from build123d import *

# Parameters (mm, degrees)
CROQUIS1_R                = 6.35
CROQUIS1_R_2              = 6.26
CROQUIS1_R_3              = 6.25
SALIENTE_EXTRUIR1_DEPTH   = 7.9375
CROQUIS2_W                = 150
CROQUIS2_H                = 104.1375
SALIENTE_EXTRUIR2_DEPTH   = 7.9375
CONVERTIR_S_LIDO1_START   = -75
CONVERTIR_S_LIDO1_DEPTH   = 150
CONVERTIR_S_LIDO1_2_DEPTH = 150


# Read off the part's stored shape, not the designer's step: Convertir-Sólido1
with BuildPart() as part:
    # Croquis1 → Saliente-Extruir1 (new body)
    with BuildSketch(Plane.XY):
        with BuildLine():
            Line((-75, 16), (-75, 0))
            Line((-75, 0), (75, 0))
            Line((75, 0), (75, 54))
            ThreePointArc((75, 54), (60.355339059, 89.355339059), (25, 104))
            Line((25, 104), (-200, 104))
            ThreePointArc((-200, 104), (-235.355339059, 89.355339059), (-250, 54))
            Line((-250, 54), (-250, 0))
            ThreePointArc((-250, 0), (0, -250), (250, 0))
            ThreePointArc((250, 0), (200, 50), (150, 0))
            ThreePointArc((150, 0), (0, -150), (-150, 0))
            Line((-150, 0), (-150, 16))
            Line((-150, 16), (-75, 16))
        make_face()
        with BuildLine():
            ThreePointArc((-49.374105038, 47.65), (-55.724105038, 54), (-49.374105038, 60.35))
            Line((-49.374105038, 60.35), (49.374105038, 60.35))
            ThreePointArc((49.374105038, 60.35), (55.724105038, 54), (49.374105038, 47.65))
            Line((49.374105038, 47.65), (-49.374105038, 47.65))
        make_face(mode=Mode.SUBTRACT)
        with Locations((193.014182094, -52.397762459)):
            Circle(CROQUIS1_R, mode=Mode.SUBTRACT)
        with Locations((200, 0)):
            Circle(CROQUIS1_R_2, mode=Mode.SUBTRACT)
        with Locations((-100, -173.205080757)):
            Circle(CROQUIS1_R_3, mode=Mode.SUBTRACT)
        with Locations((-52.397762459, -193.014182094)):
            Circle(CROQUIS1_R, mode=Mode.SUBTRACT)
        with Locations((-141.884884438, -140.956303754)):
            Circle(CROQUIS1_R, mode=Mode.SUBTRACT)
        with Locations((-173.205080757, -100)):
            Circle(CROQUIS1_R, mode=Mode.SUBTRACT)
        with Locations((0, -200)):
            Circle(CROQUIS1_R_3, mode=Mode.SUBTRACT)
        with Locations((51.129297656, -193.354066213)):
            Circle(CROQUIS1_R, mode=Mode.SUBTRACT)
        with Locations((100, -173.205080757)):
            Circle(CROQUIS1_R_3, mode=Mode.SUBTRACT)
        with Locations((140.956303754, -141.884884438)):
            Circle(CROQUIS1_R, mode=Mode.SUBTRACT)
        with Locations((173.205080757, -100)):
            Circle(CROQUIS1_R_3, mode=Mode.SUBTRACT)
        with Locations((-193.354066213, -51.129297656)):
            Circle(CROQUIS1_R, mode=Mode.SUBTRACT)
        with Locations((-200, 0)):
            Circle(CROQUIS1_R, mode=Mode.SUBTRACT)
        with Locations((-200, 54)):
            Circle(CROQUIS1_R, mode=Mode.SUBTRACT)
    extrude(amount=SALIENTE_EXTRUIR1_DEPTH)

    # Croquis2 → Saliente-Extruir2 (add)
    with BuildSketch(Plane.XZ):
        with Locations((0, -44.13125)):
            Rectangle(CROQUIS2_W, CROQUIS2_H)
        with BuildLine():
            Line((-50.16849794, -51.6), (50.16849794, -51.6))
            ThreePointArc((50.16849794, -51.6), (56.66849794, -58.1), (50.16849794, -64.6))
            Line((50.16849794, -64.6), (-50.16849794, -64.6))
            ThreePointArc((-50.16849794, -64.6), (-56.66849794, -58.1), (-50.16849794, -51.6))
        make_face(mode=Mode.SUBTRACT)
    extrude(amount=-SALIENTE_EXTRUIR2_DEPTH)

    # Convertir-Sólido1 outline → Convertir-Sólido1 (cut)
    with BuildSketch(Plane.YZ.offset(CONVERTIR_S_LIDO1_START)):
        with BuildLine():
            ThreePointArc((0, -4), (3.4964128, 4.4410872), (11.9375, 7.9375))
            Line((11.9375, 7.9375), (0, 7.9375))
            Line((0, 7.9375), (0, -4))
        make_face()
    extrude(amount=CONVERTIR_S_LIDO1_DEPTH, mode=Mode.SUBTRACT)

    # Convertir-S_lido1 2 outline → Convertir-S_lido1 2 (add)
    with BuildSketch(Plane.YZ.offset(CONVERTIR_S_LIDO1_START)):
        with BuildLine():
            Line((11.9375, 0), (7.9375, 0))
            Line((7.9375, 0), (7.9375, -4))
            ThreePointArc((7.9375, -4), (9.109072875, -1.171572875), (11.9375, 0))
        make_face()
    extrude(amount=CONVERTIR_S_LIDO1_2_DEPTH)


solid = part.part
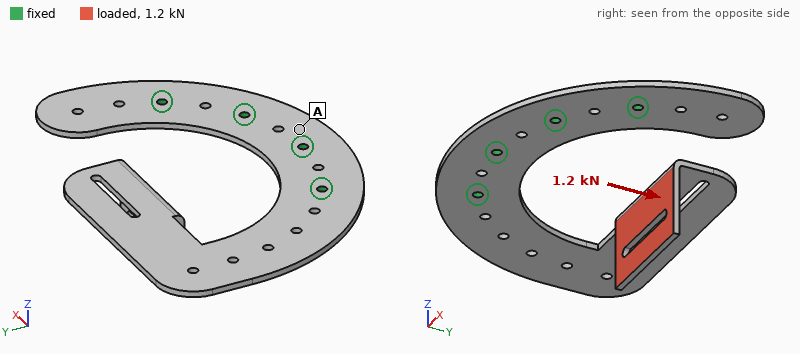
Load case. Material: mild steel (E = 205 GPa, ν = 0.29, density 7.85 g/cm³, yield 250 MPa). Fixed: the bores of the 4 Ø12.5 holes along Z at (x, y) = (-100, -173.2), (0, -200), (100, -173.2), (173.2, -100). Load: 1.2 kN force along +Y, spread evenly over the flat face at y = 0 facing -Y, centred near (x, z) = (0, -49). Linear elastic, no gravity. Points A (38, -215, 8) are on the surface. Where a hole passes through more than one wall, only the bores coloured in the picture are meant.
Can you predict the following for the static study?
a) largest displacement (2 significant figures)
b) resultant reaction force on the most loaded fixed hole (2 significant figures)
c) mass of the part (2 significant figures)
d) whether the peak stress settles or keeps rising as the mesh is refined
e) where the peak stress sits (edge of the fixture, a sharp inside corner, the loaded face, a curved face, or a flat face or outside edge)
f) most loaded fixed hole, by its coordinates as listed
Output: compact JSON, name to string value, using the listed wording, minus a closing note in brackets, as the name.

{"largest displacement": "3.4 mm", "resultant reaction force on the most loaded fixed hole": "880 N", "mass of the part": "6.7 kg", "whether the peak stress settles or keeps rising as the mesh is refined": "keeps rising", "where the peak stress sits": "a sharp inside corner", "most loaded fixed hole, by its coordinates as listed": "(0, -200)"}
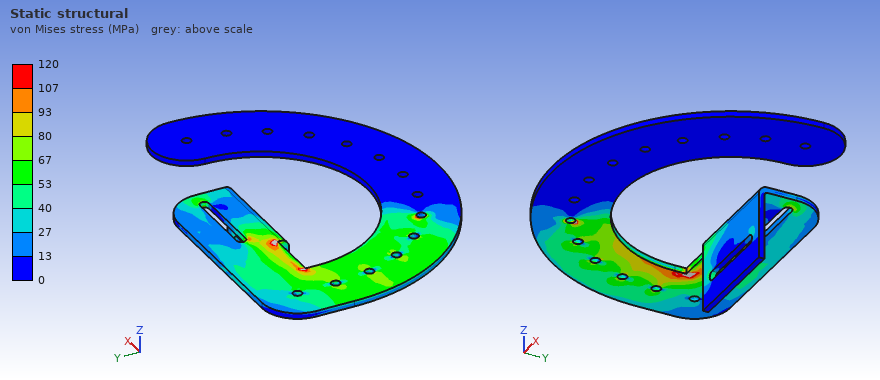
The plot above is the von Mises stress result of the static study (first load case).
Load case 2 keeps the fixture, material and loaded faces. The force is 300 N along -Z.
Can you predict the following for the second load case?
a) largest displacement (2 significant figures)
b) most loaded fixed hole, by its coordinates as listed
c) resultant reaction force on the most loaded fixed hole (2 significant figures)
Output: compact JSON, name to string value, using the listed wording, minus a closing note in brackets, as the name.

{"largest displacement": "4.4 mm", "most loaded fixed hole, by its coordinates as listed": "(-100, -173.2)", "resultant reaction force on the most loaded fixed hole": "290 N"}
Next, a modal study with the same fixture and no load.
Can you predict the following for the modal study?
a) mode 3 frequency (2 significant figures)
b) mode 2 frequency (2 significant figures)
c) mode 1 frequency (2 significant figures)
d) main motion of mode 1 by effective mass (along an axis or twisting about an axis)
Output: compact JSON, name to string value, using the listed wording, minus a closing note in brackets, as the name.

{"mode 3 frequency": "160 Hz", "mode 2 frequency": "61 Hz", "mode 1 frequency": "35 Hz", "main motion of mode 1 by effective mass": "along Z"}
